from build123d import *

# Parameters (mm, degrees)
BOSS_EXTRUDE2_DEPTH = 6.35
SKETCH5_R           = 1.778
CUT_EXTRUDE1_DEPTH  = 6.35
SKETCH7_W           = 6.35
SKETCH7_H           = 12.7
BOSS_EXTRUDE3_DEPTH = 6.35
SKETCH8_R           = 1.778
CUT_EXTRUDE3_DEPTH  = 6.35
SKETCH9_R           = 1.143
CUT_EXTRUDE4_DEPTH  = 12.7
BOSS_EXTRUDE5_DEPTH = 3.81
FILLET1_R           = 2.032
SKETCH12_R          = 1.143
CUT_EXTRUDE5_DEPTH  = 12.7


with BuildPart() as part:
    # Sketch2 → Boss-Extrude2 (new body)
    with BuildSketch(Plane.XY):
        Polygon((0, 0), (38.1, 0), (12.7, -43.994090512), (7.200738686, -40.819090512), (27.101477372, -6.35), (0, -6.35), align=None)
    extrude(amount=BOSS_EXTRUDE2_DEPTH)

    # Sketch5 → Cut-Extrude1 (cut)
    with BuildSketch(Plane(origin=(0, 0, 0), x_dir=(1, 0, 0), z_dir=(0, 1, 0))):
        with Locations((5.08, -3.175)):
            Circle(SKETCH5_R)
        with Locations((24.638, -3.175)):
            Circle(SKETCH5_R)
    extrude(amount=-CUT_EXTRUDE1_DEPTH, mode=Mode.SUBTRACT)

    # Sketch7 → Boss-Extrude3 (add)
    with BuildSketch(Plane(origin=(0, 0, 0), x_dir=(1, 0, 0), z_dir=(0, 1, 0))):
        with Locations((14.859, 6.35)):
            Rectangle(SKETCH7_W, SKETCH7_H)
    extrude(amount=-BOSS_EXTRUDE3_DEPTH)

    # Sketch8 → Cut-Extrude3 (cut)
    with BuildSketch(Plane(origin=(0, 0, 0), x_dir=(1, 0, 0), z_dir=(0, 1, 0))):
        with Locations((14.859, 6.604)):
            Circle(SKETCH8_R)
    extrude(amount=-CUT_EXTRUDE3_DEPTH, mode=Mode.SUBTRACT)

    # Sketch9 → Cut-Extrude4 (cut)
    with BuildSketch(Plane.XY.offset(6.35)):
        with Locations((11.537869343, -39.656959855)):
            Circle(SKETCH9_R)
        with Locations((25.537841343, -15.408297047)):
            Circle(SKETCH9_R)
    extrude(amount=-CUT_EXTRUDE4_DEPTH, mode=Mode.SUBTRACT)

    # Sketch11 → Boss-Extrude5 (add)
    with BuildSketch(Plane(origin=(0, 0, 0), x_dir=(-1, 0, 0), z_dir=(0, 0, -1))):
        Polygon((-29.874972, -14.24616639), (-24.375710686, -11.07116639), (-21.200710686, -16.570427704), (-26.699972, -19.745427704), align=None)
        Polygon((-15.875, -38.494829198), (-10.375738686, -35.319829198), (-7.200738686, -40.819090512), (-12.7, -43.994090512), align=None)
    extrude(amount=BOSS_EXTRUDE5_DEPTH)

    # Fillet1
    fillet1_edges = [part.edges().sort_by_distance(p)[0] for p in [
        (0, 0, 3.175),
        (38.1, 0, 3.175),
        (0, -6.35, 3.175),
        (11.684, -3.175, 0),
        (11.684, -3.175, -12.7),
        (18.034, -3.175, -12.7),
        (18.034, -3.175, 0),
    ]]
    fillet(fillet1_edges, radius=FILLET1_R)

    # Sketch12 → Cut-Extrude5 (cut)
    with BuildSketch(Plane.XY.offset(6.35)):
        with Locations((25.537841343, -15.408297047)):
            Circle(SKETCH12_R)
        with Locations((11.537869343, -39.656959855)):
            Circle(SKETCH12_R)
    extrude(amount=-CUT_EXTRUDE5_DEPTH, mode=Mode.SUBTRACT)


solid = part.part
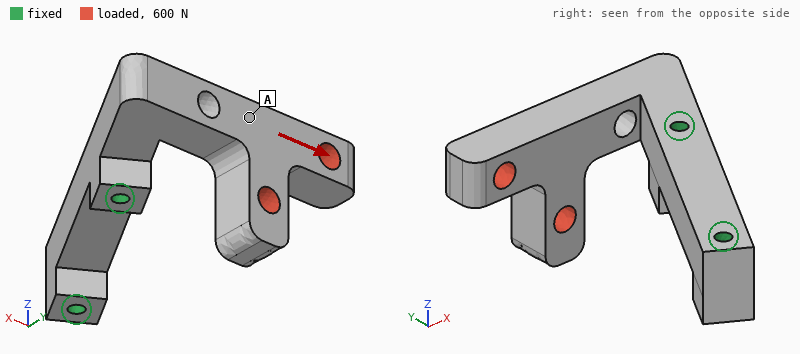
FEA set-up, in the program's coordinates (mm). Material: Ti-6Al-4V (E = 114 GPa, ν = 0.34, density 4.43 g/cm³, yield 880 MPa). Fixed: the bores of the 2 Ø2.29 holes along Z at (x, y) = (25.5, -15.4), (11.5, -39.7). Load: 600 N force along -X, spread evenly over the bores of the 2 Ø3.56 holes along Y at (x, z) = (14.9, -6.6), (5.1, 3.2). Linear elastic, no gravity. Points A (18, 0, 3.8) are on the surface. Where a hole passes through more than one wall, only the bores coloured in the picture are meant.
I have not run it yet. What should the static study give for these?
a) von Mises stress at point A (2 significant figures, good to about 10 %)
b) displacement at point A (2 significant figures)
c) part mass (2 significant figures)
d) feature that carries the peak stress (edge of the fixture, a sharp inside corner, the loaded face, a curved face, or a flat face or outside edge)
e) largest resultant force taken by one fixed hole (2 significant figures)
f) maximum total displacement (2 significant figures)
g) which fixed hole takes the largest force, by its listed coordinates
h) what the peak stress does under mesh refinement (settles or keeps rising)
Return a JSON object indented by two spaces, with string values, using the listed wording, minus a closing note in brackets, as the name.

{
  "von Mises stress at point A": "21 MPa",
  "displacement at point A": "0.074 mm",
  "part mass": "16 g",
  "feature that carries the peak stress": "edge of the fixture",
  "largest resultant force taken by one fixed hole": "660 N",
  "maximum total displacement": "0.18 mm",
  "which fixed hole takes the largest force, by its listed coordinates": "(25.5, -15.4)",
  "what the peak stress does under mesh refinement": "keeps rising"
}
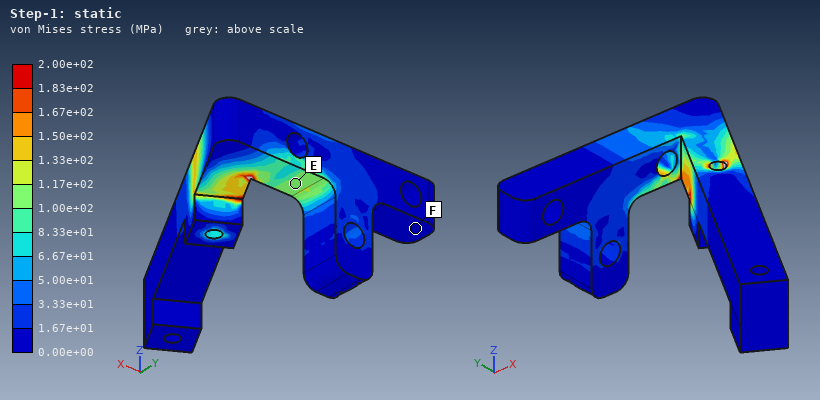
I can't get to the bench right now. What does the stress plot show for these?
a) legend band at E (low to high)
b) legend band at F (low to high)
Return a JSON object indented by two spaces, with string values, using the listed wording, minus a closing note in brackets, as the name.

{
  "legend band at E": "1.00e+02 to 1.17e+02 MPa",
  "legend band at F": "0.00e+00 to 1.67e+01 MPa"
}
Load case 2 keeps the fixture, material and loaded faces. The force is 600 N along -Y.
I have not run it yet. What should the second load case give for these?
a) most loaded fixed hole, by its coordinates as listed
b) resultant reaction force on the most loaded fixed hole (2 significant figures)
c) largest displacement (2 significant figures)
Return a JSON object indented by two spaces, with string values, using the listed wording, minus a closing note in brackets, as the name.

{
  "most loaded fixed hole, by its coordinates as listed": "(25.5, -15.4)",
  "resultant reaction force on the most loaded fixed hole": "560 N",
  "largest displacement": "0.55 mm"
}
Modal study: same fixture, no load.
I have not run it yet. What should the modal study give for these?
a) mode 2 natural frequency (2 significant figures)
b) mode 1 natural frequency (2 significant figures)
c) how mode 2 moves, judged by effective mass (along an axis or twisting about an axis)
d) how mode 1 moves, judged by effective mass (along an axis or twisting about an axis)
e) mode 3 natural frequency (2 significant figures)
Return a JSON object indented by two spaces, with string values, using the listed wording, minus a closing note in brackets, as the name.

{
  "mode 2 natural frequency": "3100 Hz",
  "mode 1 natural frequency": "2900 Hz",
  "how mode 2 moves, judged by effective mass": "along Y",
  "how mode 1 moves, judged by effective mass": "along Z",
  "mode 3 natural frequency": "6900 Hz"
}
